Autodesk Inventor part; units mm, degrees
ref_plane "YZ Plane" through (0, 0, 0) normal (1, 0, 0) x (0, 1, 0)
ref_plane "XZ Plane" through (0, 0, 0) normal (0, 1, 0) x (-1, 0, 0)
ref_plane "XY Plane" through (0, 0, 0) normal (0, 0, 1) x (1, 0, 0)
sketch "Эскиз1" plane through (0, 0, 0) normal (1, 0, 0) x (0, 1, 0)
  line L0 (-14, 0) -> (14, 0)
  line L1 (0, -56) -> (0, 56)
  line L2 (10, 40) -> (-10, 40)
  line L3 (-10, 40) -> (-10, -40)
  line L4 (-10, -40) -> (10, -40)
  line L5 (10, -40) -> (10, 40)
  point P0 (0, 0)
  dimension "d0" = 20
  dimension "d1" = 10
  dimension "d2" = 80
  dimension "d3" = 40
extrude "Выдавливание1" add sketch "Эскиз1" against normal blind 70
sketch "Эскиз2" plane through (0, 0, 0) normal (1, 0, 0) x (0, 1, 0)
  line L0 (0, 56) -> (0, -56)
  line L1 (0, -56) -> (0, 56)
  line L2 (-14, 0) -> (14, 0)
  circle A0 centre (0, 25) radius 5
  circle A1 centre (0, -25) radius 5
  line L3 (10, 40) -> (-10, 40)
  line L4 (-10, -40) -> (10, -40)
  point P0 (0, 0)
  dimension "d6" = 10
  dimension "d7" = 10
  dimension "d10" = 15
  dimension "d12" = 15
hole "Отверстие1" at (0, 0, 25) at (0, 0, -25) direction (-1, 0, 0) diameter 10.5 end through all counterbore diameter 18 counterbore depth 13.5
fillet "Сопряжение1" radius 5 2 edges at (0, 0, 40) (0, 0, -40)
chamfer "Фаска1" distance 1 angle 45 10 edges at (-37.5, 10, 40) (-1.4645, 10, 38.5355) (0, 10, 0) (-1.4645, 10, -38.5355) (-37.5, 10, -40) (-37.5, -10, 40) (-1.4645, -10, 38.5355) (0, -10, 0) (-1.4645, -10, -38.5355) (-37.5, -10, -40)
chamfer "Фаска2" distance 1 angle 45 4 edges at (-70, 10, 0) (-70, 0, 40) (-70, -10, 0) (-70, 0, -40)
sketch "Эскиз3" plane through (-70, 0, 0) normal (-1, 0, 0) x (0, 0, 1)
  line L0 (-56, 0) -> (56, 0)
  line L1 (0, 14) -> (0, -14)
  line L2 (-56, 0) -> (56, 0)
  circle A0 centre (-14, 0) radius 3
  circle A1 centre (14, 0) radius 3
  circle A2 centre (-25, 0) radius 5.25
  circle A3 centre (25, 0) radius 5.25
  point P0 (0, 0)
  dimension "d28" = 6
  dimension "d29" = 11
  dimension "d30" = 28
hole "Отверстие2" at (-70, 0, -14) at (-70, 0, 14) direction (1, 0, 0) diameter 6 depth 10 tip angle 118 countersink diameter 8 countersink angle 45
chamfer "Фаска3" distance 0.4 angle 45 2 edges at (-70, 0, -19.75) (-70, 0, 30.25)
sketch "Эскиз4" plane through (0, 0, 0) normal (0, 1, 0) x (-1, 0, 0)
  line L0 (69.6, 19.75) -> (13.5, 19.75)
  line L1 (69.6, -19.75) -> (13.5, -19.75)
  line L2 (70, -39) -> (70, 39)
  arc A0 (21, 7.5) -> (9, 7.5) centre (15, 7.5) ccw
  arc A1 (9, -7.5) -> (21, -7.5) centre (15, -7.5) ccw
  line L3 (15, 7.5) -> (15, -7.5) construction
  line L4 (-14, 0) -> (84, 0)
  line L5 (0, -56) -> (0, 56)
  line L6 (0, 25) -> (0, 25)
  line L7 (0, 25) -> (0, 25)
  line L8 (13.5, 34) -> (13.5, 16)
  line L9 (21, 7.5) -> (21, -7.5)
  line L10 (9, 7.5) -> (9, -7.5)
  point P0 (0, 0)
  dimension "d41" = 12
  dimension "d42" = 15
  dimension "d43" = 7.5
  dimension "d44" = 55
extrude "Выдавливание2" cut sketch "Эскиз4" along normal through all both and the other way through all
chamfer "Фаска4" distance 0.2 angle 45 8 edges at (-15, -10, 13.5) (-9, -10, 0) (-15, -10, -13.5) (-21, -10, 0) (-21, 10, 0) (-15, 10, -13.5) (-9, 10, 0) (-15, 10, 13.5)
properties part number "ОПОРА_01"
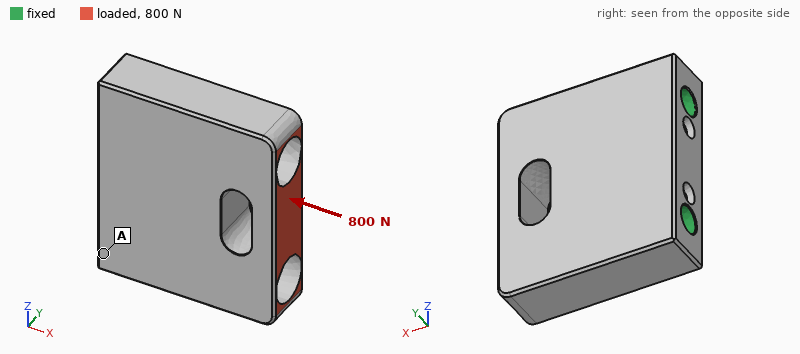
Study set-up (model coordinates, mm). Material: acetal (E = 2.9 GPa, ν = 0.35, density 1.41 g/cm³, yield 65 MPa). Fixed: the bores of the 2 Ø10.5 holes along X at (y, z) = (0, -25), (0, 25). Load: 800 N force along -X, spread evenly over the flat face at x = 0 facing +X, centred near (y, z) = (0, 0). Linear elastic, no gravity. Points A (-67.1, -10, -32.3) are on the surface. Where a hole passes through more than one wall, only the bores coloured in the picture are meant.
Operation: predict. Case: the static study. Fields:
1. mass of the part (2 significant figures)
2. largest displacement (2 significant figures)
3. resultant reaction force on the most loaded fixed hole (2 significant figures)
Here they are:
120 g
39 µm
440 N
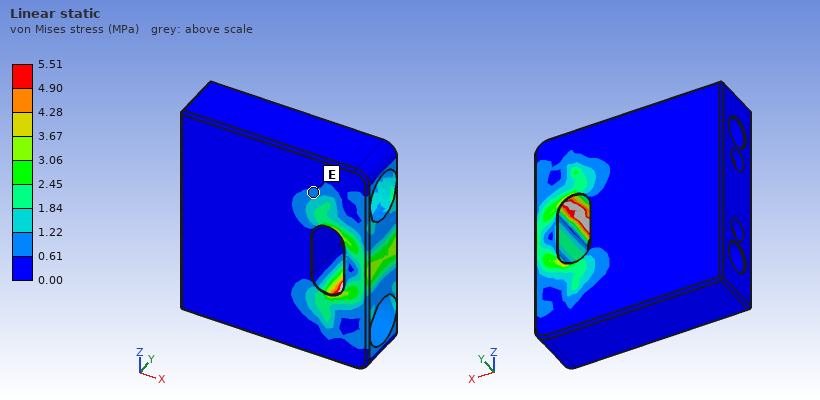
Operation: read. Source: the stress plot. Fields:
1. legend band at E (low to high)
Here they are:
0.61 to 1.22 MPa
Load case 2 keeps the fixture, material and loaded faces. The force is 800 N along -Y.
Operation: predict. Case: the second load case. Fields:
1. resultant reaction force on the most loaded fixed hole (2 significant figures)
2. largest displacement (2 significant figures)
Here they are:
400 N
0.16 mm
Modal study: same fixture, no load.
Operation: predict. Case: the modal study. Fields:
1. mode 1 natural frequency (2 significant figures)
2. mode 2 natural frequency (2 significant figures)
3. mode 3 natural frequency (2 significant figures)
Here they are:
4300 Hz
6400 Hz
6700 Hz
